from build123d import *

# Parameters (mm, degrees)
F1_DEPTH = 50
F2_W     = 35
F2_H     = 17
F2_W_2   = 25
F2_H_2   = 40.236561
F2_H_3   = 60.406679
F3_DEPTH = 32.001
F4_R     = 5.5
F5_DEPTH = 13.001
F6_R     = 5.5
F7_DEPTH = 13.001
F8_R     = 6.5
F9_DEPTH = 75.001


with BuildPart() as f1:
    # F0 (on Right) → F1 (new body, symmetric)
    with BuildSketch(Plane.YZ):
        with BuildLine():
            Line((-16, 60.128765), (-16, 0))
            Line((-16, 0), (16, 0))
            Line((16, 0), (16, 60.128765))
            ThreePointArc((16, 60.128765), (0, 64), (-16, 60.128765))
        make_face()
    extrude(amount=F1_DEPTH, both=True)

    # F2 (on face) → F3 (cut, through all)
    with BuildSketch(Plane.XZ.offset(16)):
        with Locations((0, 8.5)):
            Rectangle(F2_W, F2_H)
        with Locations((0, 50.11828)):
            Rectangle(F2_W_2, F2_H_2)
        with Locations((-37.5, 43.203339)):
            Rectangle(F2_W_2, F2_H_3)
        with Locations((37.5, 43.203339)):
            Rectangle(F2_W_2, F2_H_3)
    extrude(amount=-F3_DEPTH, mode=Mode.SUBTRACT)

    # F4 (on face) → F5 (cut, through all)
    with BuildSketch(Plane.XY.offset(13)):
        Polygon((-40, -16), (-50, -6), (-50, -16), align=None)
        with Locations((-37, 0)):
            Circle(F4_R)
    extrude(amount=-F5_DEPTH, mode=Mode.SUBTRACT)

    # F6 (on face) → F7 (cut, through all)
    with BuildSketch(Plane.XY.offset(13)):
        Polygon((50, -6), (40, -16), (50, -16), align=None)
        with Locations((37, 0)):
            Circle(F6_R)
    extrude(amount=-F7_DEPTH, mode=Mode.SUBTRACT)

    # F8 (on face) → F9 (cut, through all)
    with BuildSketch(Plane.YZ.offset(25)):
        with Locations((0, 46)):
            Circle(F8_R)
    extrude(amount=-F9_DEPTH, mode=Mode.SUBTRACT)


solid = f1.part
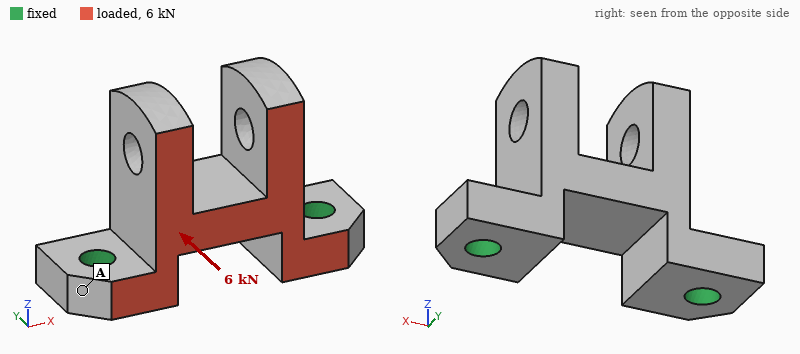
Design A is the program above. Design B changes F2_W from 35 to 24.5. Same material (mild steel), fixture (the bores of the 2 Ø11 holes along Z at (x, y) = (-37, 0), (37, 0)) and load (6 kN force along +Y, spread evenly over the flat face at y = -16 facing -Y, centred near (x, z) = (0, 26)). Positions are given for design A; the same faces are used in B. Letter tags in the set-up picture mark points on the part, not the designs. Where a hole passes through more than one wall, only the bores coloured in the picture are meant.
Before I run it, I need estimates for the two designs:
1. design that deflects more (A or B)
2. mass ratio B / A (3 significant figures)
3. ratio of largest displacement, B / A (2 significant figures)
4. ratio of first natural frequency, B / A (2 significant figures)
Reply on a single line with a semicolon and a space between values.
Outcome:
A; 1.08; 0.89; 1.0
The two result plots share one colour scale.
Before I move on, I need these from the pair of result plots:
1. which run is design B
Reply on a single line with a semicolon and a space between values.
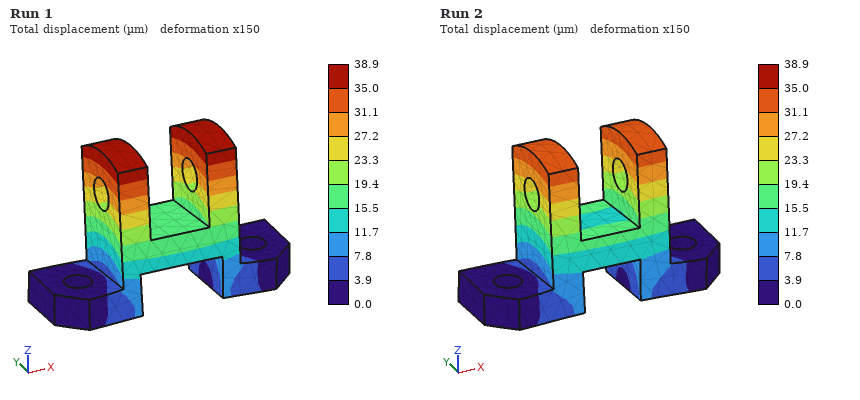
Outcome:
Run 2
